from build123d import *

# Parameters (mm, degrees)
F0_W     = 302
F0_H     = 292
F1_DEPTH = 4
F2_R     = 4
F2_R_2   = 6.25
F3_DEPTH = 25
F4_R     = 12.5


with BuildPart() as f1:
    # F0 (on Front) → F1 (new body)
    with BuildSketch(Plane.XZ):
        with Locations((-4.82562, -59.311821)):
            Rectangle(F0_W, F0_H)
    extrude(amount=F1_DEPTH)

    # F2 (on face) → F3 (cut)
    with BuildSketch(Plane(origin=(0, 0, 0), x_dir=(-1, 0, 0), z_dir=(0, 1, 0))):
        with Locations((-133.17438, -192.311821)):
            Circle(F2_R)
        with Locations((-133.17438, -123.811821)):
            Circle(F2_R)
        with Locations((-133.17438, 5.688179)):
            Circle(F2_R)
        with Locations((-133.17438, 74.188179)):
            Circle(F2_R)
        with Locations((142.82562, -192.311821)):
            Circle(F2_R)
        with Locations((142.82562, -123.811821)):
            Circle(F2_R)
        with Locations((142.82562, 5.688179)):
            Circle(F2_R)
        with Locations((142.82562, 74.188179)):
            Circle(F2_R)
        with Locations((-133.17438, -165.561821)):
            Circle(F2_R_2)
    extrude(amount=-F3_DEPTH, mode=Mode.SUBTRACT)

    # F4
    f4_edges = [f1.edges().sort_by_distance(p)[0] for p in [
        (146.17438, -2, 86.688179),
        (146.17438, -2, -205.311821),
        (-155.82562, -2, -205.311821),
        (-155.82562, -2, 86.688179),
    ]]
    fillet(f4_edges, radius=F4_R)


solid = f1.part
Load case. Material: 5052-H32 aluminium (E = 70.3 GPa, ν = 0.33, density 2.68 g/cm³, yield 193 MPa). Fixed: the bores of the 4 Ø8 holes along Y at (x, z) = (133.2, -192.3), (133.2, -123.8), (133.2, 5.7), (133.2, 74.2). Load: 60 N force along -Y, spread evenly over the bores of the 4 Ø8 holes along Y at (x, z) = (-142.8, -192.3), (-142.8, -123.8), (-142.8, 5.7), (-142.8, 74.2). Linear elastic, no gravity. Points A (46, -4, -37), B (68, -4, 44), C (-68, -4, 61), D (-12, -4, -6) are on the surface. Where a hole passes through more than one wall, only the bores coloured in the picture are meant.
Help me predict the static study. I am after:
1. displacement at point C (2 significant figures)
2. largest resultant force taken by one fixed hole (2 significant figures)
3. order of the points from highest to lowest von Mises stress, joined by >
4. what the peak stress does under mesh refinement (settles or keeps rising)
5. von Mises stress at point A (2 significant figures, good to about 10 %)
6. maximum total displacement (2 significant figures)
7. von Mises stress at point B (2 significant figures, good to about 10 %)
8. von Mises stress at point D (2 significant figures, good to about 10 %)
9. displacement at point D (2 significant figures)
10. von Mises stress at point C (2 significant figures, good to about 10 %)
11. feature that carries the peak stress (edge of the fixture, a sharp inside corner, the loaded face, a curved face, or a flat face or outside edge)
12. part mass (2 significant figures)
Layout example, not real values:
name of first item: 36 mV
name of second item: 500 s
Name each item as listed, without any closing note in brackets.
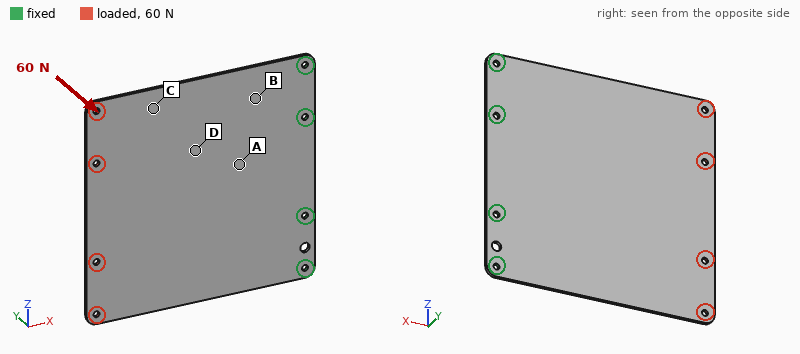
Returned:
displacement at point C: 2.4 mm
largest resultant force taken by one fixed hole: 42 N
order of the points from highest to lowest von Mises stress, joined by >: B > A > D > C
what the peak stress does under mesh refinement: keeps rising
von Mises stress at point A: 13 MPa
maximum total displacement: 4.3 mm
von Mises stress at point B: 16 MPa
von Mises stress at point D: 9.2 MPa
displacement at point D: 1.4 mm
von Mises stress at point C: 6.1 MPa
feature that carries the peak stress: edge of the fixture
part mass: 940 g
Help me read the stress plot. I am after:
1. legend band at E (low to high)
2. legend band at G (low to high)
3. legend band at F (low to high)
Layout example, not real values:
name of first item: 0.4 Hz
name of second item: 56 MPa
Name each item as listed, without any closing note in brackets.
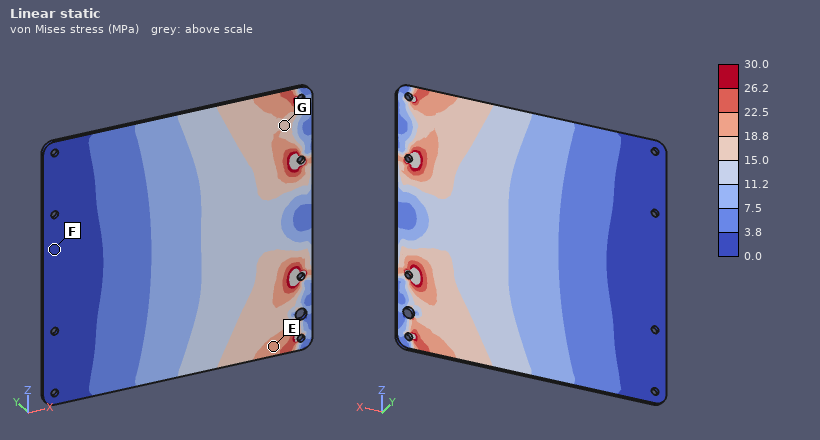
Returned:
legend band at E: 18.8 to 22.5 MPa
legend band at G: 15.0 to 18.8 MPa
legend band at F: 0.0 to 3.8 MPa
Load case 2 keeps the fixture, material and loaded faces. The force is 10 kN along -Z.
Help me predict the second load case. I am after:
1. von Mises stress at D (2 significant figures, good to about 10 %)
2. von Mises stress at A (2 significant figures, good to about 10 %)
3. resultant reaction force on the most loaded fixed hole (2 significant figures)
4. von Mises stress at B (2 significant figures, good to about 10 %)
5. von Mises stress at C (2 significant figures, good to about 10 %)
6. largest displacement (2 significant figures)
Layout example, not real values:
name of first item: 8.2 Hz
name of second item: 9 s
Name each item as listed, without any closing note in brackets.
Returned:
von Mises stress at D: 21 MPa
von Mises stress at A: 21 MPa
resultant reaction force on the most loaded fixed hole: 8.6 kN
von Mises stress at B: 28 MPa
von Mises stress at C: 13 MPa
largest displacement: 0.30 mm
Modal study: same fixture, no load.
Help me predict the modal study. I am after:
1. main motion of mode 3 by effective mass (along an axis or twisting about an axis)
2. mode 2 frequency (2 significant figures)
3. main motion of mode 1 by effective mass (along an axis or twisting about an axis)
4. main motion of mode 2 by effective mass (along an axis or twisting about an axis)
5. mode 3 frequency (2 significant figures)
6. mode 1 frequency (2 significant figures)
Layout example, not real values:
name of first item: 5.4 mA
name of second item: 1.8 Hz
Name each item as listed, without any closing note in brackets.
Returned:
main motion of mode 3 by effective mass: along Y
mode 2 frequency: 99 Hz
main motion of mode 1 by effective mass: along Y
main motion of mode 2 by effective mass: twisting about X
mode 3 frequency: 240 Hz
mode 1 frequency: 39 Hz
